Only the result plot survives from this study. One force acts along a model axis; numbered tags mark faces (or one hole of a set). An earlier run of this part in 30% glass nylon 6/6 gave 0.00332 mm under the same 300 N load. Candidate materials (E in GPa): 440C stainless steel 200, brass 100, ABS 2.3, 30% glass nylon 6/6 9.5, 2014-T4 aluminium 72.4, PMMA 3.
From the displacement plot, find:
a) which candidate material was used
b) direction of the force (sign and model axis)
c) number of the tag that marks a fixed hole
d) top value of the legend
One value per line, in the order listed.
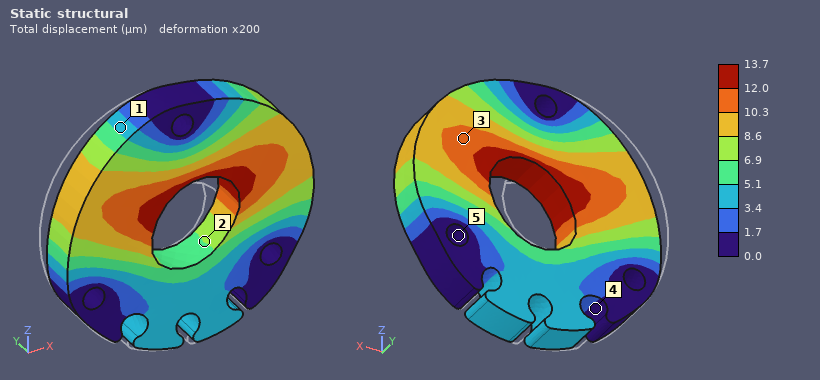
ABS
+X
5
13.7 µm
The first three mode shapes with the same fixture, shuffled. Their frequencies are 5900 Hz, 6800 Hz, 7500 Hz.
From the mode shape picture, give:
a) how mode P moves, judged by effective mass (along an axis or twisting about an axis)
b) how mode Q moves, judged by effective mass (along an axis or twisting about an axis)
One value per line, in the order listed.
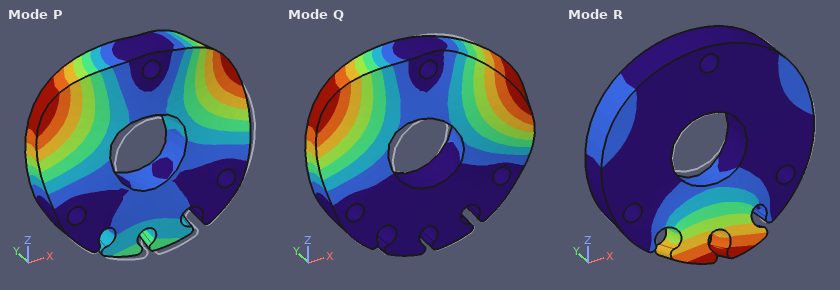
along Y
twisting about Z
